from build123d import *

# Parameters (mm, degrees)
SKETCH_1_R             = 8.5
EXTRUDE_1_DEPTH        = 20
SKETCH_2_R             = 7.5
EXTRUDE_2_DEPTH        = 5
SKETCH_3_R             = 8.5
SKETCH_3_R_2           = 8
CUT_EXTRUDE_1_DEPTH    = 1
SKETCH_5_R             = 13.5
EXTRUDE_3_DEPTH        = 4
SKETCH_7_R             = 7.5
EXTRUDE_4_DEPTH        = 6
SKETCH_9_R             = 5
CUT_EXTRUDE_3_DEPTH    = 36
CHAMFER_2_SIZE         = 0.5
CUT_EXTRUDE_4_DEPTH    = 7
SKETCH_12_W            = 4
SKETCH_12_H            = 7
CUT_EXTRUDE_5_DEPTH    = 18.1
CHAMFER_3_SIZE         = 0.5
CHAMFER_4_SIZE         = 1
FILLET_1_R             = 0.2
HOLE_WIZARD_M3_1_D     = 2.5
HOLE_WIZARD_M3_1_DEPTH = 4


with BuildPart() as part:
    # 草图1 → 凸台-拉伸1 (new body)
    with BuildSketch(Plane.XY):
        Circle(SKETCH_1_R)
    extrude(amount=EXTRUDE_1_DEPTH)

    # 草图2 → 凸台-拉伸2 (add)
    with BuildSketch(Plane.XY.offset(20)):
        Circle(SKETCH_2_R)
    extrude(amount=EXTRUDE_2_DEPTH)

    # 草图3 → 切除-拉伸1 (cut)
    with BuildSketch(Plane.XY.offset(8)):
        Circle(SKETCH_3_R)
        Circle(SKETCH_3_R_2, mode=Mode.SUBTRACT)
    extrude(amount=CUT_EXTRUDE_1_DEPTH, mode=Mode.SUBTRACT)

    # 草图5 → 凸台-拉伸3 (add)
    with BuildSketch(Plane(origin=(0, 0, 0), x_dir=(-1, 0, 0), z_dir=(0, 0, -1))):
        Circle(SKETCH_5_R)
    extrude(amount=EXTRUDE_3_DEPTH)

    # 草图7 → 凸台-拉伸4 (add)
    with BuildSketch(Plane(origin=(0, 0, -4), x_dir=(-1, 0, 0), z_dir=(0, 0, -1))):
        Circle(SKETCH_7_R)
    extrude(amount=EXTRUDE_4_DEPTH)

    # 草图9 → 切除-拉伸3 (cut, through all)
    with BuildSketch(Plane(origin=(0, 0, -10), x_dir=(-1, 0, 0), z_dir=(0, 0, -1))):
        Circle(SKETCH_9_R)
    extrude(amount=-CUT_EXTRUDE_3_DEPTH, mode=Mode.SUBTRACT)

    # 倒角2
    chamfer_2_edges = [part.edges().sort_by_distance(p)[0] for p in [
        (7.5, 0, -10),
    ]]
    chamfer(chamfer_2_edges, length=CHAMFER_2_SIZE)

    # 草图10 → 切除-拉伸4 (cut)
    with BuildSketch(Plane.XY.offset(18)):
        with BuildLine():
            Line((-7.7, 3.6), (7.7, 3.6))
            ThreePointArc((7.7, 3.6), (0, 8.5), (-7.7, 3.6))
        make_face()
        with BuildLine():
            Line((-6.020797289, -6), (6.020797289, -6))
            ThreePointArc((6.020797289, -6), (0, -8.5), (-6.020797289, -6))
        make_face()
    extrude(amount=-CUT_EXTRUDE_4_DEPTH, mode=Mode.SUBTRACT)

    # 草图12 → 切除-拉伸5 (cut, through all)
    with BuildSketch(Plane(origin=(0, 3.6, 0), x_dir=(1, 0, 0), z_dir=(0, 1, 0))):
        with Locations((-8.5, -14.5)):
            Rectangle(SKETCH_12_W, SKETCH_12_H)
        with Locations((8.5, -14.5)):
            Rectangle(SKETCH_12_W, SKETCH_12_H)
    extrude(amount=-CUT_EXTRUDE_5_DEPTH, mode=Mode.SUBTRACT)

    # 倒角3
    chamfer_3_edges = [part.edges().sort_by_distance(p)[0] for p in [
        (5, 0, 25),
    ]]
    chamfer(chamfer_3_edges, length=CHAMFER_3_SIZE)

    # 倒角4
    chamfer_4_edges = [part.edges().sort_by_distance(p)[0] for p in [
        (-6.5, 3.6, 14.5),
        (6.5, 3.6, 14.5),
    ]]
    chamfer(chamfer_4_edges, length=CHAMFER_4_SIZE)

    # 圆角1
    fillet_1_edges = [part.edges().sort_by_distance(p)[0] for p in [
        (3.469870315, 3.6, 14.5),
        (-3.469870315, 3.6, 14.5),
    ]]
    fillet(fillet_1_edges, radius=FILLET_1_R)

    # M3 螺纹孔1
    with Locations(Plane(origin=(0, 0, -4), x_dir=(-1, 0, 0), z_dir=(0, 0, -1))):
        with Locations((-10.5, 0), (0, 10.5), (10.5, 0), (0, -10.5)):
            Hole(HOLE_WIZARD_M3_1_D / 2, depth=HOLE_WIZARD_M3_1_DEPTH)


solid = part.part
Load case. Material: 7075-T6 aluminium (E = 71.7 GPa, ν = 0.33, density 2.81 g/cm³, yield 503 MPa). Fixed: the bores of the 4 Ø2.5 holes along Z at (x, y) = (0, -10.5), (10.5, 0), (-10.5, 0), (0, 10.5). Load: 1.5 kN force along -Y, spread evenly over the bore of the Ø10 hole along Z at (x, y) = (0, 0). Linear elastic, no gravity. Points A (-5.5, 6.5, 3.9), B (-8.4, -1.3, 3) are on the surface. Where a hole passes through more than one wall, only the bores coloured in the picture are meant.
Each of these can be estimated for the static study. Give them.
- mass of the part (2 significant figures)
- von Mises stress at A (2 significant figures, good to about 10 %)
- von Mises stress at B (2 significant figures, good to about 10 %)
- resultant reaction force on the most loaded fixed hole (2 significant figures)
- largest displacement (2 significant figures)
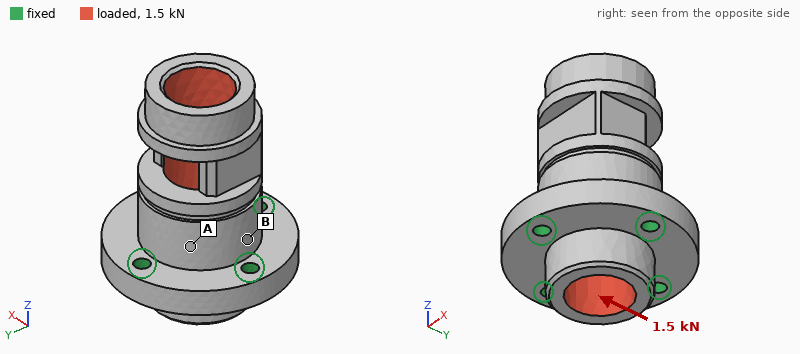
15 g
20 MPa
7.7 MPa
800 N
36 µm
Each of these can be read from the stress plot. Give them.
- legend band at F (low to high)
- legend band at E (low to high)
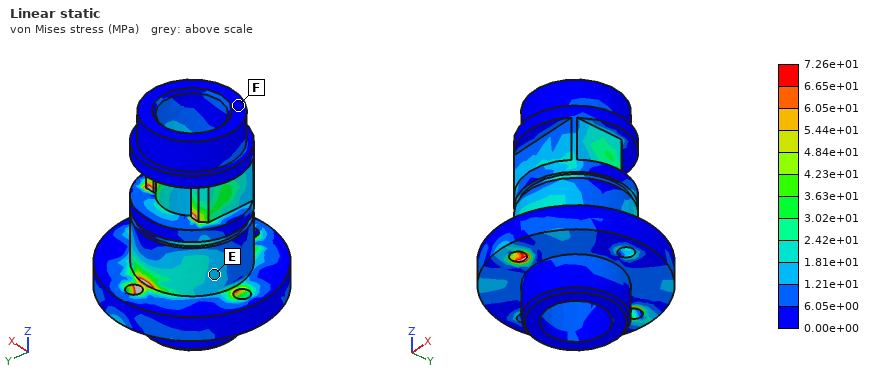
0.00e+00 to 6.05e+00 MPa
1.21e+01 to 1.81e+01 MPa
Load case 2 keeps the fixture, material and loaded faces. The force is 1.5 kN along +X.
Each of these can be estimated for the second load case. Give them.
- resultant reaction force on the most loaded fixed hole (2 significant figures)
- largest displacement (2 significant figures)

790 N
48 µm
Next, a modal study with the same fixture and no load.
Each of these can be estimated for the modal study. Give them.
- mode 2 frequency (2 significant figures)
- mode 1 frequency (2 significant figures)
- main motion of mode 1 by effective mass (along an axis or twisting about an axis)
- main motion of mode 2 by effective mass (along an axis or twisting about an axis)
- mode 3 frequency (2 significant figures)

12 kHz
11 kHz
along X
along Y
22 kHz
